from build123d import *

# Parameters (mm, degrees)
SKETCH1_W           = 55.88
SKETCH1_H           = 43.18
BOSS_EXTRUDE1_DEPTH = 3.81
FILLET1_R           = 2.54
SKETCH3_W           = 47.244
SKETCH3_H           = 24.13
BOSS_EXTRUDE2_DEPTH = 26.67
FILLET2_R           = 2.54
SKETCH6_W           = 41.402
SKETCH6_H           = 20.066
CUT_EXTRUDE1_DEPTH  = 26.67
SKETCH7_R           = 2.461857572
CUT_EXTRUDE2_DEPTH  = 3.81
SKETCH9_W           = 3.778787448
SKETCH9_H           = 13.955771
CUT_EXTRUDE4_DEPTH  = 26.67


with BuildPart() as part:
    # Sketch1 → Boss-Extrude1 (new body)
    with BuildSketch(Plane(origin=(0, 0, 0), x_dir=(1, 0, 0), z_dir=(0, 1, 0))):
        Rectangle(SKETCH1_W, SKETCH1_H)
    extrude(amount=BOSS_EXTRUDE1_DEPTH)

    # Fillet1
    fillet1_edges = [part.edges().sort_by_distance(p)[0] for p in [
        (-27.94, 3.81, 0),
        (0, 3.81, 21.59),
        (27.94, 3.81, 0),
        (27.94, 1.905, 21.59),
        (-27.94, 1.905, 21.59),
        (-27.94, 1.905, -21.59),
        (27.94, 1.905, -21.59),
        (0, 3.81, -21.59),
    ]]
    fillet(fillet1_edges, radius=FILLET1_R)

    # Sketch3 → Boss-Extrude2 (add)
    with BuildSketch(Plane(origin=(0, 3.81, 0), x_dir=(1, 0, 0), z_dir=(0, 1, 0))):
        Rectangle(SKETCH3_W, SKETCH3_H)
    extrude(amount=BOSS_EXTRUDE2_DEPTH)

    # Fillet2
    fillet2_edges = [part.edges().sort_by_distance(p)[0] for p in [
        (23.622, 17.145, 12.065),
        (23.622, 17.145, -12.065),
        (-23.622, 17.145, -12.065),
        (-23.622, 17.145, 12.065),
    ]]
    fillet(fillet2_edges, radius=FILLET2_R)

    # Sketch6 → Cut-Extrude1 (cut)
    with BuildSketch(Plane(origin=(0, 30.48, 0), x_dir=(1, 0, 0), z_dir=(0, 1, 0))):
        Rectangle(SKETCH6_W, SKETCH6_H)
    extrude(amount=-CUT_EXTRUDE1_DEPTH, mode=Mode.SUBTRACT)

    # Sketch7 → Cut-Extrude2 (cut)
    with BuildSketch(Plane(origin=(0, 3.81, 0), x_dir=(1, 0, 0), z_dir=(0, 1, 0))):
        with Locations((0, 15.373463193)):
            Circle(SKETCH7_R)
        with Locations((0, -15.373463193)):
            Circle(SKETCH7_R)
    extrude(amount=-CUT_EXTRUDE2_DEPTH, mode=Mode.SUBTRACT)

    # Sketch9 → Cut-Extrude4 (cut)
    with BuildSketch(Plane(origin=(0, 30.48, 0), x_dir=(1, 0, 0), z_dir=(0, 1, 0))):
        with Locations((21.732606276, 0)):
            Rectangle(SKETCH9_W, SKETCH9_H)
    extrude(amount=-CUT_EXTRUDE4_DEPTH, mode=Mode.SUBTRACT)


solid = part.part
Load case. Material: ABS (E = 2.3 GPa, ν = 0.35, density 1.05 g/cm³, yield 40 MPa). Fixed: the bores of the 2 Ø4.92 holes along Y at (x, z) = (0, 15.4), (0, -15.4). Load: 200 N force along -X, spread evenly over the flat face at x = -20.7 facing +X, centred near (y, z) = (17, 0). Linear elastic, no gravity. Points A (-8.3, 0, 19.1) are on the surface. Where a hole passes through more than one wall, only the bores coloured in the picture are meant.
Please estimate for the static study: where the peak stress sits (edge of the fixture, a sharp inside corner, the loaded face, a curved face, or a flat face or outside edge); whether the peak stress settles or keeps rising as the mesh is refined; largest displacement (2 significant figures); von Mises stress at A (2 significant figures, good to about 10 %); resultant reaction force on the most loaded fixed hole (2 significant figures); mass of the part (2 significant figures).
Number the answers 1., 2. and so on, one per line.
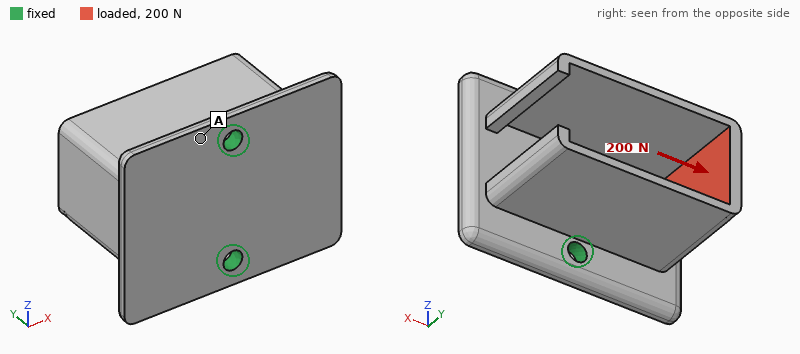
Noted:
1. edge of the fixture
2. keeps rising
3. 0.80 mm
4. 5.0 MPa
5. 100 N
6. 17 g
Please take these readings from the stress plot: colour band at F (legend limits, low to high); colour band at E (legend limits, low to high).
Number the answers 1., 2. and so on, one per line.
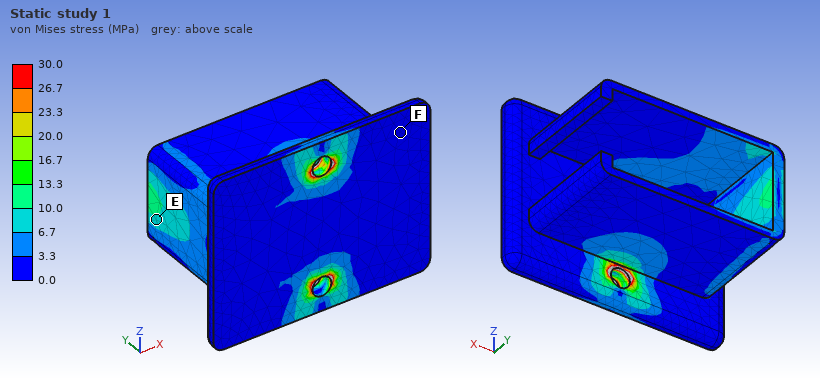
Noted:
1. 0.0 to 3.3 MPa
2. 6.7 to 10.0 MPa
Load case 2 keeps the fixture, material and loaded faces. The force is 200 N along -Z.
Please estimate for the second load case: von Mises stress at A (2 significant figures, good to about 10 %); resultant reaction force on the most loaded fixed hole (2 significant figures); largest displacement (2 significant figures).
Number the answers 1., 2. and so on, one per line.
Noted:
1. 6.2 MPa
2. 190 N
3. 0.74 mm
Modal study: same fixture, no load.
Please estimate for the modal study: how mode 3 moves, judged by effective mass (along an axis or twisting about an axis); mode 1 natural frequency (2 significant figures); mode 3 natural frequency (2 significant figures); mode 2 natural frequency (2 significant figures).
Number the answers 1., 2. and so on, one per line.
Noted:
1. along Z
2. 860 Hz
3. 1200 Hz
4. 1000 Hz
